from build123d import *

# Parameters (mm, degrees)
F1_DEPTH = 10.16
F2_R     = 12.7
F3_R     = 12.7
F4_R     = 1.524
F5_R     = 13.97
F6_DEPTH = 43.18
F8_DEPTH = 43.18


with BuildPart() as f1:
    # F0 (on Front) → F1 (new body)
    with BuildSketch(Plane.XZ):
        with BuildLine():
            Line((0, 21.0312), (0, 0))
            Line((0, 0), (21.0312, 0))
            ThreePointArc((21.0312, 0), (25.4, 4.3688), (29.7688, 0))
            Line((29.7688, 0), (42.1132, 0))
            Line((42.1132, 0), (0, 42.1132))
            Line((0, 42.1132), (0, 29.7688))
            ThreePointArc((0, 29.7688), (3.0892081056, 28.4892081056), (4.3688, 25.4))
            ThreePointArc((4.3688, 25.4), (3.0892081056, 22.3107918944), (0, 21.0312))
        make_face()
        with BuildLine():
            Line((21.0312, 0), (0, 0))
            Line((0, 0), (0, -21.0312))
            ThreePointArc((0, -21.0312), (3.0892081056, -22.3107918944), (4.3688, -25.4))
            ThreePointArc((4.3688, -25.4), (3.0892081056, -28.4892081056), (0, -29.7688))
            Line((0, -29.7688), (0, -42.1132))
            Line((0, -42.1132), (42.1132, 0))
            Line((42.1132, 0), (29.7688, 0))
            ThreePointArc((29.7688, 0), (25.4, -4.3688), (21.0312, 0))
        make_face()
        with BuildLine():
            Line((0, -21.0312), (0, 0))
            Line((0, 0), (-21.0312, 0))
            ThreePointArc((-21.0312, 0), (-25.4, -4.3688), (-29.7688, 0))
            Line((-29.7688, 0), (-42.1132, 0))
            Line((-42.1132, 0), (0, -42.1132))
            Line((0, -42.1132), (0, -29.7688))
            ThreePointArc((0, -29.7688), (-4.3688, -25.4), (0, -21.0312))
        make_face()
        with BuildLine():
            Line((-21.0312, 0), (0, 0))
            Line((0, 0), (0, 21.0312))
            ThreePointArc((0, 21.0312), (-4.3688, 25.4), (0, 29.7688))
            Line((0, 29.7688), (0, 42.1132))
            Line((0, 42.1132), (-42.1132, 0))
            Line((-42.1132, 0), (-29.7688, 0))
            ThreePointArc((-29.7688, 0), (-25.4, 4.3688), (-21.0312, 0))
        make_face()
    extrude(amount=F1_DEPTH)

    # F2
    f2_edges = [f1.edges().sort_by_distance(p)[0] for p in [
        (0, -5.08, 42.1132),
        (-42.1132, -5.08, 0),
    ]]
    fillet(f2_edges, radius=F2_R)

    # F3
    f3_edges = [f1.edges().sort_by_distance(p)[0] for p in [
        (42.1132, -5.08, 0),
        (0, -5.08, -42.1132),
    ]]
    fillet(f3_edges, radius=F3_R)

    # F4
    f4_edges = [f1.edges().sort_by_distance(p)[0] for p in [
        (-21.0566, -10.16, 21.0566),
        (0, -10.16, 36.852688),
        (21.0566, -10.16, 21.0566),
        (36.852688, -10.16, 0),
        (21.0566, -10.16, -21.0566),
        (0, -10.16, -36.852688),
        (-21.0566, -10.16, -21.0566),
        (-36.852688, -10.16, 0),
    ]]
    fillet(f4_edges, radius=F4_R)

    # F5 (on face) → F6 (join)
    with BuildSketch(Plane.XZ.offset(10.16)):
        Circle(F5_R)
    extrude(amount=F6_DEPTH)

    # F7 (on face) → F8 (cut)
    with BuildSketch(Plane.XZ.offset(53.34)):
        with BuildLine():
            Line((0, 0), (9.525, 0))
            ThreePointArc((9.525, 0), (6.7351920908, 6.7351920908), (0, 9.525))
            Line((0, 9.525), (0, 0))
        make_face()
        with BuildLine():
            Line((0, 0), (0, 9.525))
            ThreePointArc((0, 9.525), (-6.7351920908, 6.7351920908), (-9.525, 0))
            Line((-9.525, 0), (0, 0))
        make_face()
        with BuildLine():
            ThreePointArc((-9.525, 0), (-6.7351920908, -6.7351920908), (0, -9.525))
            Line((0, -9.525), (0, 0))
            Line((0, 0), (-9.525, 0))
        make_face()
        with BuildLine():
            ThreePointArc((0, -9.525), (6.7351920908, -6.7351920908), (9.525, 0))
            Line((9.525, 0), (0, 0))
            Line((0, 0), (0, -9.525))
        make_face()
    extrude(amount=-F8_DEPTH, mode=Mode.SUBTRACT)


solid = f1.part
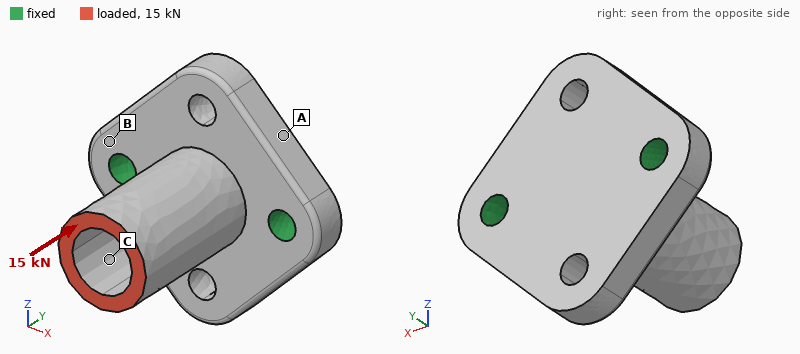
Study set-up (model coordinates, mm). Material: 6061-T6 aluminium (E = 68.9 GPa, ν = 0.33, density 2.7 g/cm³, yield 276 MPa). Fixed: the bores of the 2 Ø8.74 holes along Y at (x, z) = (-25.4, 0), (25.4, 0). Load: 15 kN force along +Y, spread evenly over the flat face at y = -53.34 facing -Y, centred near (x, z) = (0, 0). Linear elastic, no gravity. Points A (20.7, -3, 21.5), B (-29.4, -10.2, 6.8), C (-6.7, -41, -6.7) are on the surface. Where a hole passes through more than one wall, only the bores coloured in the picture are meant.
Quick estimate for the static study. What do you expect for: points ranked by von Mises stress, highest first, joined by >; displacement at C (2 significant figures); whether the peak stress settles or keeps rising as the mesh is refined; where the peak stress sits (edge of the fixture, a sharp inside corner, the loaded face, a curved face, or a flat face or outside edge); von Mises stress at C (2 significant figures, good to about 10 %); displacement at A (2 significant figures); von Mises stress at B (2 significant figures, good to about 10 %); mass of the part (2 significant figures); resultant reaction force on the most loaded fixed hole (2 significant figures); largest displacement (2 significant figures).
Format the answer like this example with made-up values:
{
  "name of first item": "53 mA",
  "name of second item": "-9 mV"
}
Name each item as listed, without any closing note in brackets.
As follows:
{
  "points ranked by von Mises stress, highest first, joined by >": "C > B > A",
  "displacement at C": "52 µm",
  "whether the peak stress settles or keeps rising as the mesh is refined": "keeps rising",
  "where the peak stress sits": "edge of the fixture",
  "von Mises stress at C": "46 MPa",
  "displacement at A": "20 µm",
  "von Mises stress at B": "31 MPa",
  "mass of the part": "120 g",
  "resultant reaction force on the most loaded fixed hole": "7.6 kN",
  "largest displacement": "61 µm"
}
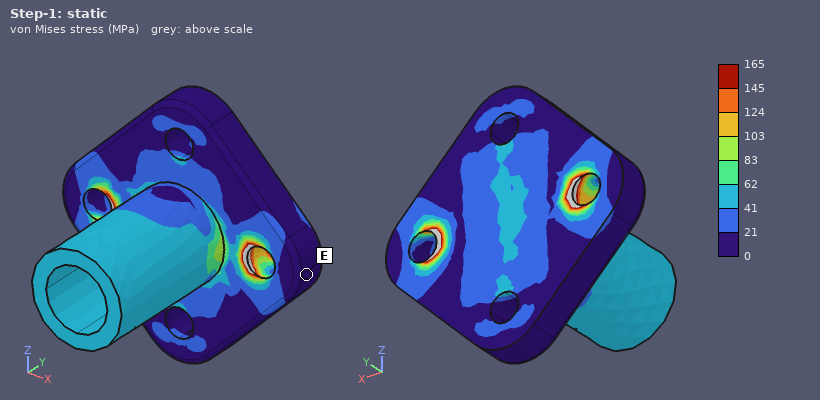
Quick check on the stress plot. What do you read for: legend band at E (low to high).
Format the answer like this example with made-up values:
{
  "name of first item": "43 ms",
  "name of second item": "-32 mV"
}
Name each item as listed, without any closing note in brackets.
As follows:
{
  "legend band at E": "0 to 21 MPa"
}
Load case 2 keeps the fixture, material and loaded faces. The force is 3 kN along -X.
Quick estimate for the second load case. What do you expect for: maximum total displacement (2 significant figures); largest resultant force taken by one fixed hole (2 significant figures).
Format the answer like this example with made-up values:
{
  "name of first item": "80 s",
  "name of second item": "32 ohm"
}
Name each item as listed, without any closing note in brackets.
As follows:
{
  "maximum total displacement": "0.13 mm",
  "largest resultant force taken by one fixed hole": "4.0 kN"
}
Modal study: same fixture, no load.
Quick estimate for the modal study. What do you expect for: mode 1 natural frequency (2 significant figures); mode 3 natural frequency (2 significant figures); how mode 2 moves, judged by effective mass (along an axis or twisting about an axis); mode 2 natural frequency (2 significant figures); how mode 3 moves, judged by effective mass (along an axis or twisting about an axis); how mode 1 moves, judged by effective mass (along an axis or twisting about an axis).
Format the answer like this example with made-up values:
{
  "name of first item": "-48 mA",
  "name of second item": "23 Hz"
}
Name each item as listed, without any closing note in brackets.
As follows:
{
  "mode 1 natural frequency": "4200 Hz",
  "mode 3 natural frequency": "9000 Hz",
  "how mode 2 moves, judged by effective mass": "along X",
  "mode 2 natural frequency": "7200 Hz",
  "how mode 3 moves, judged by effective mass": "along Y",
  "how mode 1 moves, judged by effective mass": "along Z"
}
